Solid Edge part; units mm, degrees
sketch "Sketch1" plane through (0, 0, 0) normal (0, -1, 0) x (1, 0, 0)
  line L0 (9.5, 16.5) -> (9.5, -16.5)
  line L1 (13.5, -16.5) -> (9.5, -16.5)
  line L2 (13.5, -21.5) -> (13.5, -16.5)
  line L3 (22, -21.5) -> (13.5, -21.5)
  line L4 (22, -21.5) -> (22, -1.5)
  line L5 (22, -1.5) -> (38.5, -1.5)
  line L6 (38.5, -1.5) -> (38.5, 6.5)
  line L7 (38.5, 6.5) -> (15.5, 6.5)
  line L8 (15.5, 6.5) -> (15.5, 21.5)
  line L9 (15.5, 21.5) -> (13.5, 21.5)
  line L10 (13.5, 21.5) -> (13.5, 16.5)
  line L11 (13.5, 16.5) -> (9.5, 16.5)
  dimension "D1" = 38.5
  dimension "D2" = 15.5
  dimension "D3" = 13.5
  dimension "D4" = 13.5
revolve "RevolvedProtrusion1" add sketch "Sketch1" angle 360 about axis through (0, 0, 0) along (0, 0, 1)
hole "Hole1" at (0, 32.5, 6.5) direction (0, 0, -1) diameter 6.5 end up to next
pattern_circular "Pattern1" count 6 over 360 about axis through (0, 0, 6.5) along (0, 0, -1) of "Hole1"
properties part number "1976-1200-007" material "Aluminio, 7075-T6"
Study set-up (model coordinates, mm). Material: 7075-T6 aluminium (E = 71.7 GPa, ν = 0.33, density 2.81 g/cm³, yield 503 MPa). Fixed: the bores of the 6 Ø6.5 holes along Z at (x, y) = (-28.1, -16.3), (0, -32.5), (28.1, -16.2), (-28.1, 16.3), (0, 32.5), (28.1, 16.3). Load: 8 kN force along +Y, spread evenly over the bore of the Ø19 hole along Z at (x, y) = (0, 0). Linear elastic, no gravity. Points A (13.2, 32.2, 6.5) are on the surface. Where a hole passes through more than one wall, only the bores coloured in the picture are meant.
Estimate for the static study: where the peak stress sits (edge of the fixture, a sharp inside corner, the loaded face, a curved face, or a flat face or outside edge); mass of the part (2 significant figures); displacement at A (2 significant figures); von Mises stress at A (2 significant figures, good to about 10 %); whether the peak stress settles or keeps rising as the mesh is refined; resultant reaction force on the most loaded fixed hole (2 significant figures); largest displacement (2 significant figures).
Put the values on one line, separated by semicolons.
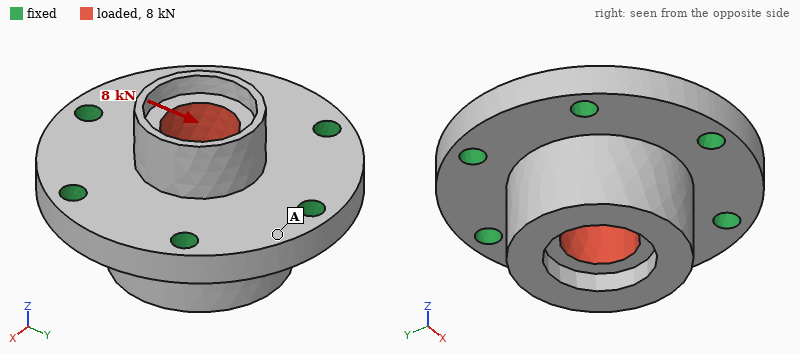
edge of the fixture; 180 g; 1.8 µm; 4.3 MPa; keeps rising; 2.0 kN; 6.0 µm
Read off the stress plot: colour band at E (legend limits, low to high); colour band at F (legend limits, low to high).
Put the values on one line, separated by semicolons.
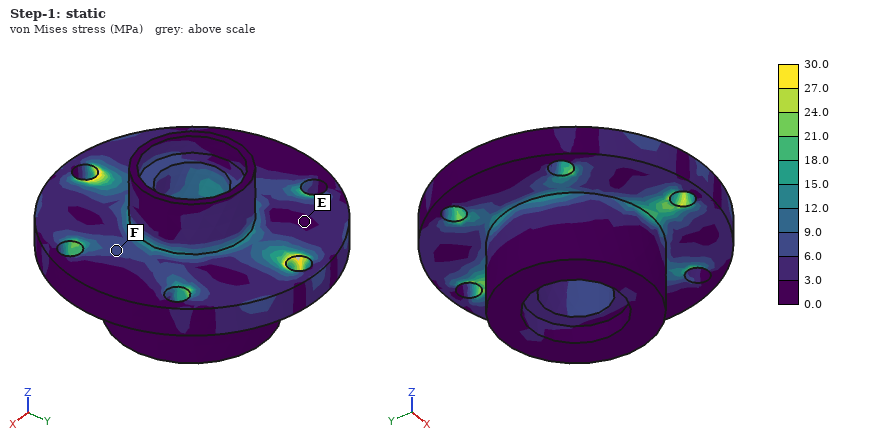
0.0 to 3.0 MPa; 6.0 to 9.0 MPa
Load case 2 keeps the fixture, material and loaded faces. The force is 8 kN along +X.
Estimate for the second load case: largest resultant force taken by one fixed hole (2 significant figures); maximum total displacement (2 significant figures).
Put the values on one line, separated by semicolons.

1.7 kN; 6.0 µm
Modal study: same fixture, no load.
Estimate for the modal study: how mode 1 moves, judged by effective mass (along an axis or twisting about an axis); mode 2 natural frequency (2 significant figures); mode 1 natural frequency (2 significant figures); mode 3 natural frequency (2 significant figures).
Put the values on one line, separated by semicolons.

along Z; 15 kHz; 14 kHz; 16 kHz
